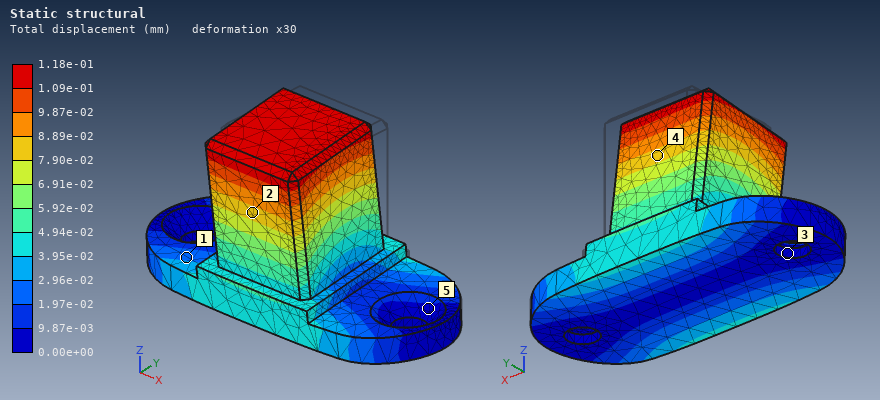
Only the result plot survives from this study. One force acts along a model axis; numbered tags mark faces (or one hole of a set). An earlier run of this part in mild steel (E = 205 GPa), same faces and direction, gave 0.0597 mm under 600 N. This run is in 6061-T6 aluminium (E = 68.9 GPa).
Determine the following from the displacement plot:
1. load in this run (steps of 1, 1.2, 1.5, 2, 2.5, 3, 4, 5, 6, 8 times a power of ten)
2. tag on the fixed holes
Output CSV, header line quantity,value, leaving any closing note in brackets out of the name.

quantity,value
load in this run,400 N
tag on the fixed holes,3
